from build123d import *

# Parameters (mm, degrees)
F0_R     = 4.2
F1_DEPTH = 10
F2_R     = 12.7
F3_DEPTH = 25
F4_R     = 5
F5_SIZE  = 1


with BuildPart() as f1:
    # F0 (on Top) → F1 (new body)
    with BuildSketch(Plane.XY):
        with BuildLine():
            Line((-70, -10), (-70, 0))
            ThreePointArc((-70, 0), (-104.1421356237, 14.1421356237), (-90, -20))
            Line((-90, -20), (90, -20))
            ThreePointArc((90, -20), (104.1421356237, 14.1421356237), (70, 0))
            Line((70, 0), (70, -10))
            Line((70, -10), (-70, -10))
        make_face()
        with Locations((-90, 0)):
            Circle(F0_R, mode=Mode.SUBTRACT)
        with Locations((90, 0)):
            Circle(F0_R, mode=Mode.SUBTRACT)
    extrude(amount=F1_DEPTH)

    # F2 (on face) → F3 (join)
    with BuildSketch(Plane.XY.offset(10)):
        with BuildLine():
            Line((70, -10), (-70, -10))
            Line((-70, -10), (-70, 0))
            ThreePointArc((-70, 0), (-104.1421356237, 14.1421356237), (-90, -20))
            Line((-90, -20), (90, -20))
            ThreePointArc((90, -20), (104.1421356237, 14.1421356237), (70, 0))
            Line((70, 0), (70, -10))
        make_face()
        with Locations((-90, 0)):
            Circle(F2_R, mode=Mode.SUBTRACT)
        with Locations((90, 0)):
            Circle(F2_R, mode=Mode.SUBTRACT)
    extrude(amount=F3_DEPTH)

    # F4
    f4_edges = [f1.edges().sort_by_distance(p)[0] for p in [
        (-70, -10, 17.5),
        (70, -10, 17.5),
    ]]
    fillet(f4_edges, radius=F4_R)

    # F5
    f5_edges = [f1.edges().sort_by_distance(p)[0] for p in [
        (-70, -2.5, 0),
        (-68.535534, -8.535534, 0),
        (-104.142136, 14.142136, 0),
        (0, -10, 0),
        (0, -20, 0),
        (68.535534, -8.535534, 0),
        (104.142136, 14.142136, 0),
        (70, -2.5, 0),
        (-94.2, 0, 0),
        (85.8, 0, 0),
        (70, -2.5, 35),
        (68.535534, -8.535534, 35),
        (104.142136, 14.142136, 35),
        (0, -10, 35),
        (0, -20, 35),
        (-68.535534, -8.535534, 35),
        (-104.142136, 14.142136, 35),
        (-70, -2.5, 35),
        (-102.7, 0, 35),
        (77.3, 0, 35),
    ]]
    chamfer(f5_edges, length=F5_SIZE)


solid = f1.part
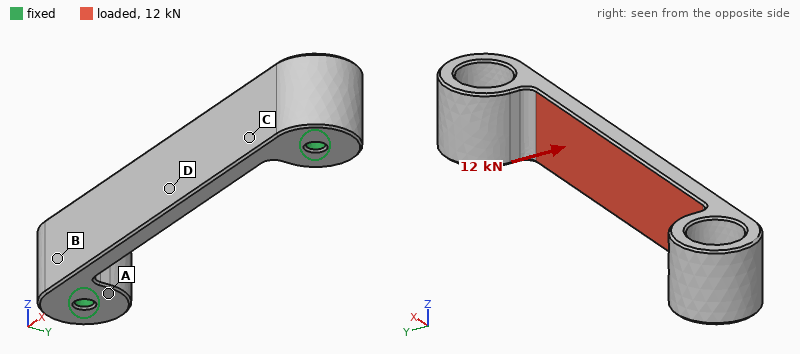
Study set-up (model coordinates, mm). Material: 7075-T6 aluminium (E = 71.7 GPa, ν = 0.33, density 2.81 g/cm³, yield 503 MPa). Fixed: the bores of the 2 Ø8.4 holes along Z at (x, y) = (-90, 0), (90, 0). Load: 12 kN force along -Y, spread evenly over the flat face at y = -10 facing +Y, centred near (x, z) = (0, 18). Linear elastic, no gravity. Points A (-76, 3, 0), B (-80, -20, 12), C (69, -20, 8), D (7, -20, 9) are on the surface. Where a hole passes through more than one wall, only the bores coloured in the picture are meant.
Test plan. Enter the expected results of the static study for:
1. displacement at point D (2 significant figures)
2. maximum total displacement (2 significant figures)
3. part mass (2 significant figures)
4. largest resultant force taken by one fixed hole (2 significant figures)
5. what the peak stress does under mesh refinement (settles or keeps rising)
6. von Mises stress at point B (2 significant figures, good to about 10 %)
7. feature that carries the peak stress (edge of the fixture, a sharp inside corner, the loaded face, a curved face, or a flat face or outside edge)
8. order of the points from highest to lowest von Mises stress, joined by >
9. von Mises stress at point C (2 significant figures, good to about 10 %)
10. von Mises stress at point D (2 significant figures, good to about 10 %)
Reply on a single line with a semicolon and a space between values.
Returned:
0.71 mm; 0.80 mm; 330 g; 9.4 kN; keeps rising; 69 MPa; edge of the fixture; D > C > B > A; 140 MPa; 180 MPa
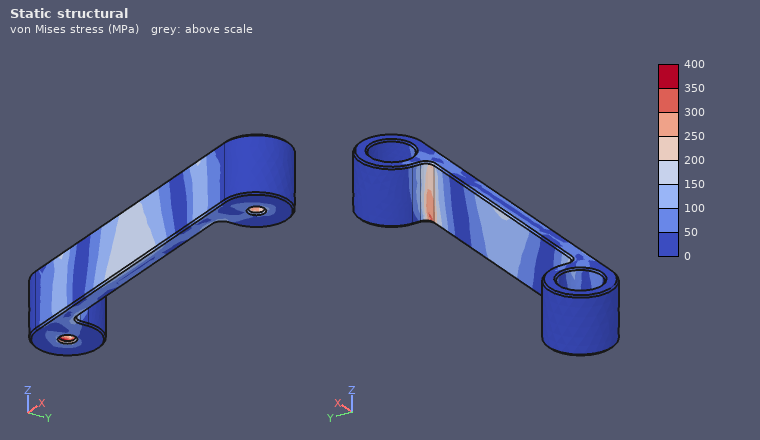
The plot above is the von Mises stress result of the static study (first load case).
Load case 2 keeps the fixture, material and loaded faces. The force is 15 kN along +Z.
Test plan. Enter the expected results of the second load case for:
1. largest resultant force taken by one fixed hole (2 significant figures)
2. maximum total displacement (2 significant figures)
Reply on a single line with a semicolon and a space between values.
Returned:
9.2 kN; 0.37 mm
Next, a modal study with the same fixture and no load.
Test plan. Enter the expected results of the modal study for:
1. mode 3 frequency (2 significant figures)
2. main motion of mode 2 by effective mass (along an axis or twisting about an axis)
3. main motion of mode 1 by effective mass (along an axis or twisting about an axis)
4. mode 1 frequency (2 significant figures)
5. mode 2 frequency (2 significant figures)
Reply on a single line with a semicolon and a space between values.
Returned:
4000 Hz; along Z; along Y; 2000 Hz; 3200 Hz
